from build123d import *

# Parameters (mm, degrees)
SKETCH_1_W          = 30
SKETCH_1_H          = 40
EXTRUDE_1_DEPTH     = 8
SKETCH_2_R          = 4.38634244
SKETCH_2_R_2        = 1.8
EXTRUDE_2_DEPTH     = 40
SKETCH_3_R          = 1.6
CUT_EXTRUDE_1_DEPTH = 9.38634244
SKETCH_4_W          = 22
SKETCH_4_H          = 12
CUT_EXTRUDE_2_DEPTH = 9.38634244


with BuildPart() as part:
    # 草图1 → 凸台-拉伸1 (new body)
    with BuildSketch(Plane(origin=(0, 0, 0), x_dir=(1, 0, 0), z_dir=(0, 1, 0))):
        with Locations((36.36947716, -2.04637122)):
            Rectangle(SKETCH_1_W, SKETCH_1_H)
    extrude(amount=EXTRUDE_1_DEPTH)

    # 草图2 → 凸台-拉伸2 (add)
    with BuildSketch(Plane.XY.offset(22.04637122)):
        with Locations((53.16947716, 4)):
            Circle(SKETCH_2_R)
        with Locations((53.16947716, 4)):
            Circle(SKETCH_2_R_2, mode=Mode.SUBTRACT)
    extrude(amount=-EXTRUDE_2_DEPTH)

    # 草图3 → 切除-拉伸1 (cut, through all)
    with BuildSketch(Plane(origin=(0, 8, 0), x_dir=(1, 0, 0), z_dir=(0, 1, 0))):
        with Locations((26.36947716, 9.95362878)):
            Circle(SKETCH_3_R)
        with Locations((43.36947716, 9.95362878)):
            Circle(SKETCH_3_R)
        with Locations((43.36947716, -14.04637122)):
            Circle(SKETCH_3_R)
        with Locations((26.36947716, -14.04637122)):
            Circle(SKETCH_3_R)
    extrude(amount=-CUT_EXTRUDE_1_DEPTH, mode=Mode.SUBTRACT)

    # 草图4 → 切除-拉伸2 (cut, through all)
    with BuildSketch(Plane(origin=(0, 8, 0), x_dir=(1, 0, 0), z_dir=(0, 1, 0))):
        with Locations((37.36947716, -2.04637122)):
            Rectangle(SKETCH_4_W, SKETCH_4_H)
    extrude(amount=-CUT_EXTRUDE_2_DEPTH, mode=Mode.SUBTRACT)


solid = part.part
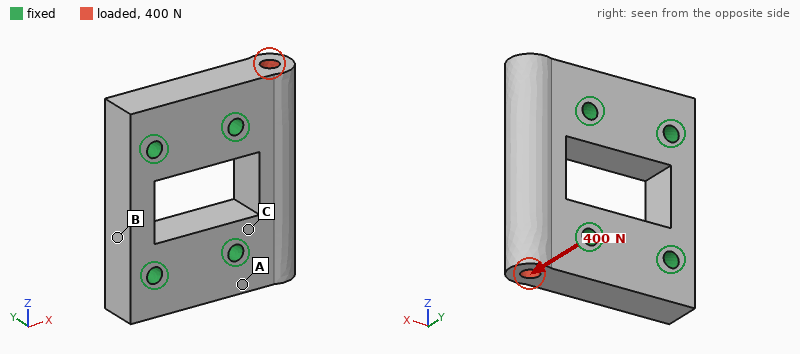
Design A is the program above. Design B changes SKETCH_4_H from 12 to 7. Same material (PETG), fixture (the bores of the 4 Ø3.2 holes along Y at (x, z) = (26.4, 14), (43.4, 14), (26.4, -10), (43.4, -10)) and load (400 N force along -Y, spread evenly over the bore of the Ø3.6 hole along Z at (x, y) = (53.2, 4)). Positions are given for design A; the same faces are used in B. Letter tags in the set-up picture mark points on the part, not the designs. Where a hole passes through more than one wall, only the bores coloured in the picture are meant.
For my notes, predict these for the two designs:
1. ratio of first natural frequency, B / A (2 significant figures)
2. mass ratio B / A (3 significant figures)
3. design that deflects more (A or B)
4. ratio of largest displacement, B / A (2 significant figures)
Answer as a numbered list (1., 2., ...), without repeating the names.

1. 1.0
2. 1.10
3. A
4. 0.89
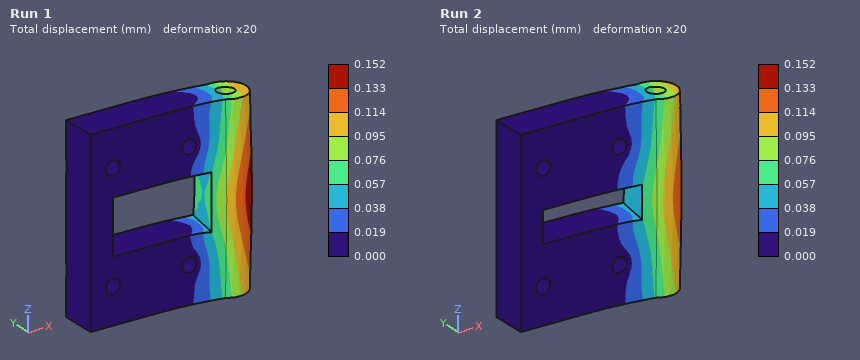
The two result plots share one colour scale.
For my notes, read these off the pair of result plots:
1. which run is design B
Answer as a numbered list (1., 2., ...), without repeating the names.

1. Run 2
